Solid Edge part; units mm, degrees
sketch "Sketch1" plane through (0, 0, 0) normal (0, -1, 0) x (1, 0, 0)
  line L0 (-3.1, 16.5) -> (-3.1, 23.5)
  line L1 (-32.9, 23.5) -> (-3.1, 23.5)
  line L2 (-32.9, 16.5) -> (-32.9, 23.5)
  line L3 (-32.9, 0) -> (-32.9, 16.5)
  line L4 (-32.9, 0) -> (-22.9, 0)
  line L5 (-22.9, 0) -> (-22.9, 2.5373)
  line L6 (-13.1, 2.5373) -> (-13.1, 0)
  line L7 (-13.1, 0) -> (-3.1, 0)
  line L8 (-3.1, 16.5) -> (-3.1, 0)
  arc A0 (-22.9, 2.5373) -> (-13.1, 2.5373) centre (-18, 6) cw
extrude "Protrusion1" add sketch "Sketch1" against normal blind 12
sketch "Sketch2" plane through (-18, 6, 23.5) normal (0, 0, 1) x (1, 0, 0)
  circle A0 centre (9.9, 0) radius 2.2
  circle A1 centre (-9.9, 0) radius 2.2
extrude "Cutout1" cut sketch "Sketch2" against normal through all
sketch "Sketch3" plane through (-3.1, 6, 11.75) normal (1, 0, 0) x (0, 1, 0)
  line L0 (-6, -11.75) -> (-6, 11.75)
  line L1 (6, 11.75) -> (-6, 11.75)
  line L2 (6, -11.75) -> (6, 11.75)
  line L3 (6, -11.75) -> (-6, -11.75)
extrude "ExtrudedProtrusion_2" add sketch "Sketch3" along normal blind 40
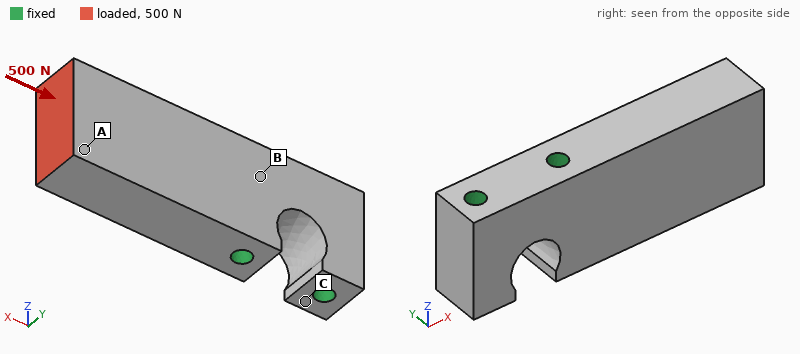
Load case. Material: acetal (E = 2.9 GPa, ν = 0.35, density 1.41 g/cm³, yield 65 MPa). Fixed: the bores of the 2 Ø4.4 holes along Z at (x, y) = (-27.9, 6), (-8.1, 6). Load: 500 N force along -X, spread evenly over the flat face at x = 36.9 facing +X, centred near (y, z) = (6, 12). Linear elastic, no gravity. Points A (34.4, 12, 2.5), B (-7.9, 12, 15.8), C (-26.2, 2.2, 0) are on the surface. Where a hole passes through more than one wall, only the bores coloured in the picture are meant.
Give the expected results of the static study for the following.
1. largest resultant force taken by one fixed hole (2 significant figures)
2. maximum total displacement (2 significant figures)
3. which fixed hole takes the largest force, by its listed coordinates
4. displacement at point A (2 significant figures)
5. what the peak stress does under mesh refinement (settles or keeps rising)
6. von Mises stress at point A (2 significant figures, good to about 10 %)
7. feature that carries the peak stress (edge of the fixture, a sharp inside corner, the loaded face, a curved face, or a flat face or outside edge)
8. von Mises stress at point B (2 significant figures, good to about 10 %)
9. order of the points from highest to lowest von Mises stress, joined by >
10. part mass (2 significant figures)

480 N
28 µm
(-8.1, 6)
26 µm
keeps rising
1.8 MPa
edge of the fixture
0.88 MPa
A > B > C
25 g
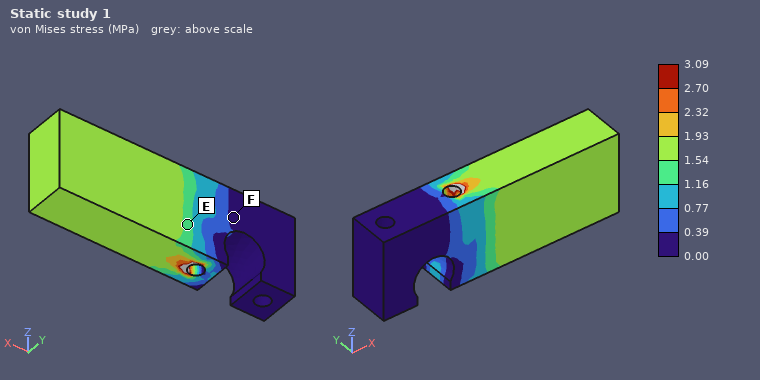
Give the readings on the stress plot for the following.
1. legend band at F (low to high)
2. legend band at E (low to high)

0.00 to 0.39 MPa
1.16 to 1.54 MPa
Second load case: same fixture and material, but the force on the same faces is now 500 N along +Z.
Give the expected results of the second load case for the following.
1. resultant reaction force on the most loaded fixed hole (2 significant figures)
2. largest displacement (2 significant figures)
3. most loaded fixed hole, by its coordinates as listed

540 N
0.52 mm
(-8.1, 6)
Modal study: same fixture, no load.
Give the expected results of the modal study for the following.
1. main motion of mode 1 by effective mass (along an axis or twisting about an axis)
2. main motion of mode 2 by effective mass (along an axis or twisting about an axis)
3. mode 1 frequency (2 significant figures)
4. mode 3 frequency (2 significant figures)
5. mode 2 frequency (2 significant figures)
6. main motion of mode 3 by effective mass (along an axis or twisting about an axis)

along Y
along Z
1200 Hz
3800 Hz
2300 Hz
twisting about X
